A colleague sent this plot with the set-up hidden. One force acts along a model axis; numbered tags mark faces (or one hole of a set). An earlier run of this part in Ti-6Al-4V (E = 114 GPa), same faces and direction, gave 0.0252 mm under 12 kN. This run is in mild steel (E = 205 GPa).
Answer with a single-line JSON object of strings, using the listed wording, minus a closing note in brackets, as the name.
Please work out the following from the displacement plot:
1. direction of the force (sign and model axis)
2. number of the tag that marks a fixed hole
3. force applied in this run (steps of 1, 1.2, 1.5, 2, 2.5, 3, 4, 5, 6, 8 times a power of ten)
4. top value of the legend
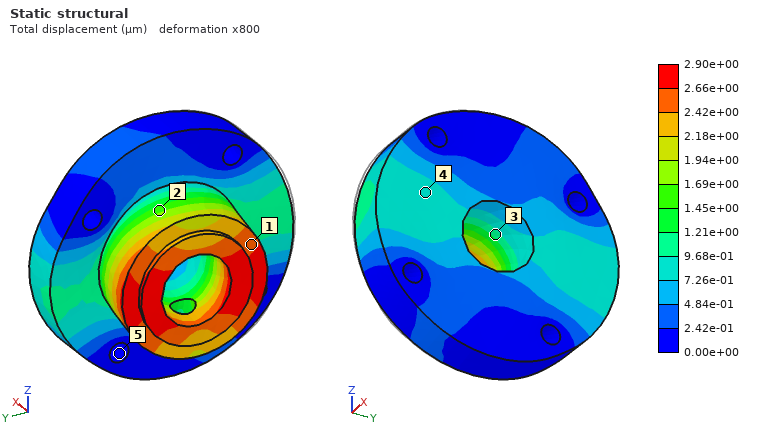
{"direction of the force": "+Y", "number of the tag that marks a fixed hole": "5", "force applied in this run": "2.5 kN", "top value of the legend": "2.90e+00 µm"}
